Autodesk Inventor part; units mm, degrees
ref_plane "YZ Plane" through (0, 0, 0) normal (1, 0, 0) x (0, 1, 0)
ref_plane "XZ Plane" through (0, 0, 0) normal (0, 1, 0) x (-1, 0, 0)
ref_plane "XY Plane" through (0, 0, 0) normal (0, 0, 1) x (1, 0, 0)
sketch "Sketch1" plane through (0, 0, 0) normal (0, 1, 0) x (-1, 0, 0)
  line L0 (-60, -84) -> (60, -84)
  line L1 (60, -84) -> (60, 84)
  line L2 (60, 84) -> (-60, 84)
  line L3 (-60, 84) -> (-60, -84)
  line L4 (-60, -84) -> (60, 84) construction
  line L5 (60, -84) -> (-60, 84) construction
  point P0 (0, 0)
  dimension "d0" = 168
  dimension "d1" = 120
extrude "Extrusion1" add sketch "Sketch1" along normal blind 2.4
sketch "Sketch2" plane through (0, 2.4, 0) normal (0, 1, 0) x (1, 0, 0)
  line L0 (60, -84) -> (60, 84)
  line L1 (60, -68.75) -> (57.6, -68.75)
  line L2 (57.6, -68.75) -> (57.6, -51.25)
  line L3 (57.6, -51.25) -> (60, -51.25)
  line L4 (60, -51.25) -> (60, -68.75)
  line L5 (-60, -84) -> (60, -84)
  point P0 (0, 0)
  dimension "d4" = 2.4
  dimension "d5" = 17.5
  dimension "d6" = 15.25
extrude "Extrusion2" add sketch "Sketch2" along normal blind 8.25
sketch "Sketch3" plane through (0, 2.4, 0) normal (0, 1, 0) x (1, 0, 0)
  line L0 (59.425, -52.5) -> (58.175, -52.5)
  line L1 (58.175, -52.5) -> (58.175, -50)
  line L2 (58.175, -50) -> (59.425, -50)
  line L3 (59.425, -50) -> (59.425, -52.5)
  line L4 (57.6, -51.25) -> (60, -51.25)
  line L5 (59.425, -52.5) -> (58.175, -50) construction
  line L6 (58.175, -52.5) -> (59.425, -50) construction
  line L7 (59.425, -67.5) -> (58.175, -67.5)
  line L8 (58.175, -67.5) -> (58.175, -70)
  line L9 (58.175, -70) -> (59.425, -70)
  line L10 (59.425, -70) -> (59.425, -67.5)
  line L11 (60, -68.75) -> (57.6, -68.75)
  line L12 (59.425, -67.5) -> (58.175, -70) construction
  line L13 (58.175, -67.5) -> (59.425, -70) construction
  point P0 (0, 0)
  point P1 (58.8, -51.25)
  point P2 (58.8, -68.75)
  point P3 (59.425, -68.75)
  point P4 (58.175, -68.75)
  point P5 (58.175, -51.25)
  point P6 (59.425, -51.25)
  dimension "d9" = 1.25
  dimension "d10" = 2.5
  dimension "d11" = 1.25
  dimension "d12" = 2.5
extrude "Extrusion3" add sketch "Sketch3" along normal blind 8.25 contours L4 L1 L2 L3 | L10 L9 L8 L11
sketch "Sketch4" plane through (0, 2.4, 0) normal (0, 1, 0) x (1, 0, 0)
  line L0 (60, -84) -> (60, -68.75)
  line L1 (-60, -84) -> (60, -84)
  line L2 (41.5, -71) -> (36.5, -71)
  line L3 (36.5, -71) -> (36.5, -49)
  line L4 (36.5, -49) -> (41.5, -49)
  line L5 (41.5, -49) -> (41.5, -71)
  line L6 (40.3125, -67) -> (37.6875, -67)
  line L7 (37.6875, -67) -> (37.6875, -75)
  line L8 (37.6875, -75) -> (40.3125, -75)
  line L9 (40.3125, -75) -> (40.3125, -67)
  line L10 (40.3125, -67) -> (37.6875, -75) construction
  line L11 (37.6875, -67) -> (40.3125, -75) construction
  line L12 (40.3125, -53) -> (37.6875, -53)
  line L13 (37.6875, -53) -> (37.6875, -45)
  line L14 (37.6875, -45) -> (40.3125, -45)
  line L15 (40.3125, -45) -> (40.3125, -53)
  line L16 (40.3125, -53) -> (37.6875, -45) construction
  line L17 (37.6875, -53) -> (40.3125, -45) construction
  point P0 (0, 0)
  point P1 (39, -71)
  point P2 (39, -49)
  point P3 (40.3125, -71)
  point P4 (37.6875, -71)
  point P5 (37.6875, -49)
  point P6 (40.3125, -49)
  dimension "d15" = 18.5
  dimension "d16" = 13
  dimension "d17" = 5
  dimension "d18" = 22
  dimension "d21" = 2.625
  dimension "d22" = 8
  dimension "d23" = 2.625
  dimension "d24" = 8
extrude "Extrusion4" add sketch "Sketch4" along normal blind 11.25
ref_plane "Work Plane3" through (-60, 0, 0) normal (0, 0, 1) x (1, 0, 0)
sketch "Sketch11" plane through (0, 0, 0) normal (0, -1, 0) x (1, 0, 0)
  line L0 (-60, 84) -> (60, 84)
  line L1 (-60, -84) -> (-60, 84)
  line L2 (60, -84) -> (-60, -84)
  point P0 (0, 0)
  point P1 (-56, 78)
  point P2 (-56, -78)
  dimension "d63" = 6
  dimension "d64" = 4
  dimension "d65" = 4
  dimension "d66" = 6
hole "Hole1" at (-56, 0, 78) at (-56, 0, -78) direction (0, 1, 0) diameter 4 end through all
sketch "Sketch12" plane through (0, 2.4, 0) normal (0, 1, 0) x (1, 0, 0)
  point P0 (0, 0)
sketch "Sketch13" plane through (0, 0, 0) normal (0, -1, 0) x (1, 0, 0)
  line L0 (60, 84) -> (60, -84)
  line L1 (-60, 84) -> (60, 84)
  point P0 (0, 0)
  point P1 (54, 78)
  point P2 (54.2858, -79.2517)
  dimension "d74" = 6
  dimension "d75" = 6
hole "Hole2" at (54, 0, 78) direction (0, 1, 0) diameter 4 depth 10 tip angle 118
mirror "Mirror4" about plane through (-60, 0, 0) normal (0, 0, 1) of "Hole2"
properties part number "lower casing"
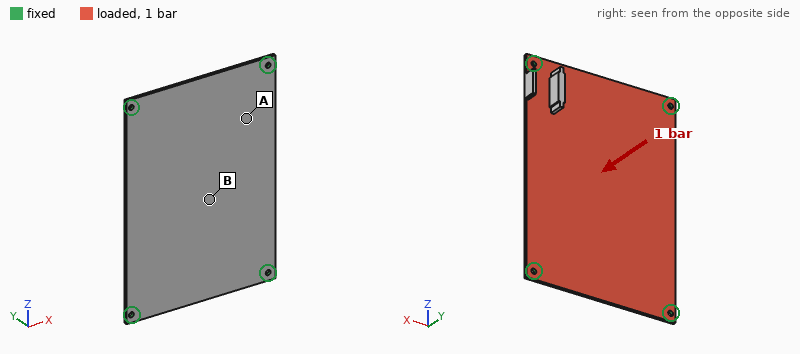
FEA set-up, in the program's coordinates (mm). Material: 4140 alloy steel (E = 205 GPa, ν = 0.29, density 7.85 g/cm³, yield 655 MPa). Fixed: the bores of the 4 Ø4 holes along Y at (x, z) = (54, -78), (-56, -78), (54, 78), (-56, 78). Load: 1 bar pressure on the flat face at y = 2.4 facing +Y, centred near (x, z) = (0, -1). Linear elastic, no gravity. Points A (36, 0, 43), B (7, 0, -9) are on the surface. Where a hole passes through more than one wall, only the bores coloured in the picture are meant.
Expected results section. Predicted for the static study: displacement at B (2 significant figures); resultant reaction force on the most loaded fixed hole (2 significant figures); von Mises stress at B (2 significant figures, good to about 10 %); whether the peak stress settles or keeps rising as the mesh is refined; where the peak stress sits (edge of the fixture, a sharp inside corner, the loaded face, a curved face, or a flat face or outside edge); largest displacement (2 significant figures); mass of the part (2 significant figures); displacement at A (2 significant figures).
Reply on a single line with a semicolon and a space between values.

1.2 mm; 520 N; 120 MPa; keeps rising; edge of the fixture; 1.2 mm; 390 g; 0.65 mm
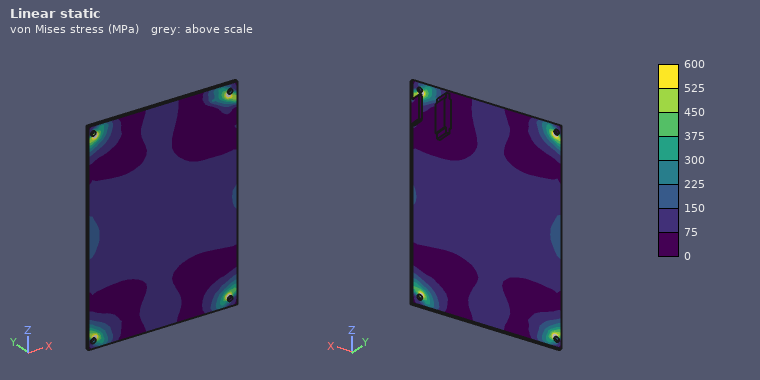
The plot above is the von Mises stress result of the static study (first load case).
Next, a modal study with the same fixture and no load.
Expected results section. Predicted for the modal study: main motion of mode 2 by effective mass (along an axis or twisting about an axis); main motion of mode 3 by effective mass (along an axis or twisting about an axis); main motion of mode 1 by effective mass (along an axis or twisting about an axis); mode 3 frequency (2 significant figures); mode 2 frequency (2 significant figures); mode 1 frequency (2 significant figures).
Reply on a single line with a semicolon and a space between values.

twisting about Z; twisting about X; along Y; 900 Hz; 670 Hz; 380 Hz
